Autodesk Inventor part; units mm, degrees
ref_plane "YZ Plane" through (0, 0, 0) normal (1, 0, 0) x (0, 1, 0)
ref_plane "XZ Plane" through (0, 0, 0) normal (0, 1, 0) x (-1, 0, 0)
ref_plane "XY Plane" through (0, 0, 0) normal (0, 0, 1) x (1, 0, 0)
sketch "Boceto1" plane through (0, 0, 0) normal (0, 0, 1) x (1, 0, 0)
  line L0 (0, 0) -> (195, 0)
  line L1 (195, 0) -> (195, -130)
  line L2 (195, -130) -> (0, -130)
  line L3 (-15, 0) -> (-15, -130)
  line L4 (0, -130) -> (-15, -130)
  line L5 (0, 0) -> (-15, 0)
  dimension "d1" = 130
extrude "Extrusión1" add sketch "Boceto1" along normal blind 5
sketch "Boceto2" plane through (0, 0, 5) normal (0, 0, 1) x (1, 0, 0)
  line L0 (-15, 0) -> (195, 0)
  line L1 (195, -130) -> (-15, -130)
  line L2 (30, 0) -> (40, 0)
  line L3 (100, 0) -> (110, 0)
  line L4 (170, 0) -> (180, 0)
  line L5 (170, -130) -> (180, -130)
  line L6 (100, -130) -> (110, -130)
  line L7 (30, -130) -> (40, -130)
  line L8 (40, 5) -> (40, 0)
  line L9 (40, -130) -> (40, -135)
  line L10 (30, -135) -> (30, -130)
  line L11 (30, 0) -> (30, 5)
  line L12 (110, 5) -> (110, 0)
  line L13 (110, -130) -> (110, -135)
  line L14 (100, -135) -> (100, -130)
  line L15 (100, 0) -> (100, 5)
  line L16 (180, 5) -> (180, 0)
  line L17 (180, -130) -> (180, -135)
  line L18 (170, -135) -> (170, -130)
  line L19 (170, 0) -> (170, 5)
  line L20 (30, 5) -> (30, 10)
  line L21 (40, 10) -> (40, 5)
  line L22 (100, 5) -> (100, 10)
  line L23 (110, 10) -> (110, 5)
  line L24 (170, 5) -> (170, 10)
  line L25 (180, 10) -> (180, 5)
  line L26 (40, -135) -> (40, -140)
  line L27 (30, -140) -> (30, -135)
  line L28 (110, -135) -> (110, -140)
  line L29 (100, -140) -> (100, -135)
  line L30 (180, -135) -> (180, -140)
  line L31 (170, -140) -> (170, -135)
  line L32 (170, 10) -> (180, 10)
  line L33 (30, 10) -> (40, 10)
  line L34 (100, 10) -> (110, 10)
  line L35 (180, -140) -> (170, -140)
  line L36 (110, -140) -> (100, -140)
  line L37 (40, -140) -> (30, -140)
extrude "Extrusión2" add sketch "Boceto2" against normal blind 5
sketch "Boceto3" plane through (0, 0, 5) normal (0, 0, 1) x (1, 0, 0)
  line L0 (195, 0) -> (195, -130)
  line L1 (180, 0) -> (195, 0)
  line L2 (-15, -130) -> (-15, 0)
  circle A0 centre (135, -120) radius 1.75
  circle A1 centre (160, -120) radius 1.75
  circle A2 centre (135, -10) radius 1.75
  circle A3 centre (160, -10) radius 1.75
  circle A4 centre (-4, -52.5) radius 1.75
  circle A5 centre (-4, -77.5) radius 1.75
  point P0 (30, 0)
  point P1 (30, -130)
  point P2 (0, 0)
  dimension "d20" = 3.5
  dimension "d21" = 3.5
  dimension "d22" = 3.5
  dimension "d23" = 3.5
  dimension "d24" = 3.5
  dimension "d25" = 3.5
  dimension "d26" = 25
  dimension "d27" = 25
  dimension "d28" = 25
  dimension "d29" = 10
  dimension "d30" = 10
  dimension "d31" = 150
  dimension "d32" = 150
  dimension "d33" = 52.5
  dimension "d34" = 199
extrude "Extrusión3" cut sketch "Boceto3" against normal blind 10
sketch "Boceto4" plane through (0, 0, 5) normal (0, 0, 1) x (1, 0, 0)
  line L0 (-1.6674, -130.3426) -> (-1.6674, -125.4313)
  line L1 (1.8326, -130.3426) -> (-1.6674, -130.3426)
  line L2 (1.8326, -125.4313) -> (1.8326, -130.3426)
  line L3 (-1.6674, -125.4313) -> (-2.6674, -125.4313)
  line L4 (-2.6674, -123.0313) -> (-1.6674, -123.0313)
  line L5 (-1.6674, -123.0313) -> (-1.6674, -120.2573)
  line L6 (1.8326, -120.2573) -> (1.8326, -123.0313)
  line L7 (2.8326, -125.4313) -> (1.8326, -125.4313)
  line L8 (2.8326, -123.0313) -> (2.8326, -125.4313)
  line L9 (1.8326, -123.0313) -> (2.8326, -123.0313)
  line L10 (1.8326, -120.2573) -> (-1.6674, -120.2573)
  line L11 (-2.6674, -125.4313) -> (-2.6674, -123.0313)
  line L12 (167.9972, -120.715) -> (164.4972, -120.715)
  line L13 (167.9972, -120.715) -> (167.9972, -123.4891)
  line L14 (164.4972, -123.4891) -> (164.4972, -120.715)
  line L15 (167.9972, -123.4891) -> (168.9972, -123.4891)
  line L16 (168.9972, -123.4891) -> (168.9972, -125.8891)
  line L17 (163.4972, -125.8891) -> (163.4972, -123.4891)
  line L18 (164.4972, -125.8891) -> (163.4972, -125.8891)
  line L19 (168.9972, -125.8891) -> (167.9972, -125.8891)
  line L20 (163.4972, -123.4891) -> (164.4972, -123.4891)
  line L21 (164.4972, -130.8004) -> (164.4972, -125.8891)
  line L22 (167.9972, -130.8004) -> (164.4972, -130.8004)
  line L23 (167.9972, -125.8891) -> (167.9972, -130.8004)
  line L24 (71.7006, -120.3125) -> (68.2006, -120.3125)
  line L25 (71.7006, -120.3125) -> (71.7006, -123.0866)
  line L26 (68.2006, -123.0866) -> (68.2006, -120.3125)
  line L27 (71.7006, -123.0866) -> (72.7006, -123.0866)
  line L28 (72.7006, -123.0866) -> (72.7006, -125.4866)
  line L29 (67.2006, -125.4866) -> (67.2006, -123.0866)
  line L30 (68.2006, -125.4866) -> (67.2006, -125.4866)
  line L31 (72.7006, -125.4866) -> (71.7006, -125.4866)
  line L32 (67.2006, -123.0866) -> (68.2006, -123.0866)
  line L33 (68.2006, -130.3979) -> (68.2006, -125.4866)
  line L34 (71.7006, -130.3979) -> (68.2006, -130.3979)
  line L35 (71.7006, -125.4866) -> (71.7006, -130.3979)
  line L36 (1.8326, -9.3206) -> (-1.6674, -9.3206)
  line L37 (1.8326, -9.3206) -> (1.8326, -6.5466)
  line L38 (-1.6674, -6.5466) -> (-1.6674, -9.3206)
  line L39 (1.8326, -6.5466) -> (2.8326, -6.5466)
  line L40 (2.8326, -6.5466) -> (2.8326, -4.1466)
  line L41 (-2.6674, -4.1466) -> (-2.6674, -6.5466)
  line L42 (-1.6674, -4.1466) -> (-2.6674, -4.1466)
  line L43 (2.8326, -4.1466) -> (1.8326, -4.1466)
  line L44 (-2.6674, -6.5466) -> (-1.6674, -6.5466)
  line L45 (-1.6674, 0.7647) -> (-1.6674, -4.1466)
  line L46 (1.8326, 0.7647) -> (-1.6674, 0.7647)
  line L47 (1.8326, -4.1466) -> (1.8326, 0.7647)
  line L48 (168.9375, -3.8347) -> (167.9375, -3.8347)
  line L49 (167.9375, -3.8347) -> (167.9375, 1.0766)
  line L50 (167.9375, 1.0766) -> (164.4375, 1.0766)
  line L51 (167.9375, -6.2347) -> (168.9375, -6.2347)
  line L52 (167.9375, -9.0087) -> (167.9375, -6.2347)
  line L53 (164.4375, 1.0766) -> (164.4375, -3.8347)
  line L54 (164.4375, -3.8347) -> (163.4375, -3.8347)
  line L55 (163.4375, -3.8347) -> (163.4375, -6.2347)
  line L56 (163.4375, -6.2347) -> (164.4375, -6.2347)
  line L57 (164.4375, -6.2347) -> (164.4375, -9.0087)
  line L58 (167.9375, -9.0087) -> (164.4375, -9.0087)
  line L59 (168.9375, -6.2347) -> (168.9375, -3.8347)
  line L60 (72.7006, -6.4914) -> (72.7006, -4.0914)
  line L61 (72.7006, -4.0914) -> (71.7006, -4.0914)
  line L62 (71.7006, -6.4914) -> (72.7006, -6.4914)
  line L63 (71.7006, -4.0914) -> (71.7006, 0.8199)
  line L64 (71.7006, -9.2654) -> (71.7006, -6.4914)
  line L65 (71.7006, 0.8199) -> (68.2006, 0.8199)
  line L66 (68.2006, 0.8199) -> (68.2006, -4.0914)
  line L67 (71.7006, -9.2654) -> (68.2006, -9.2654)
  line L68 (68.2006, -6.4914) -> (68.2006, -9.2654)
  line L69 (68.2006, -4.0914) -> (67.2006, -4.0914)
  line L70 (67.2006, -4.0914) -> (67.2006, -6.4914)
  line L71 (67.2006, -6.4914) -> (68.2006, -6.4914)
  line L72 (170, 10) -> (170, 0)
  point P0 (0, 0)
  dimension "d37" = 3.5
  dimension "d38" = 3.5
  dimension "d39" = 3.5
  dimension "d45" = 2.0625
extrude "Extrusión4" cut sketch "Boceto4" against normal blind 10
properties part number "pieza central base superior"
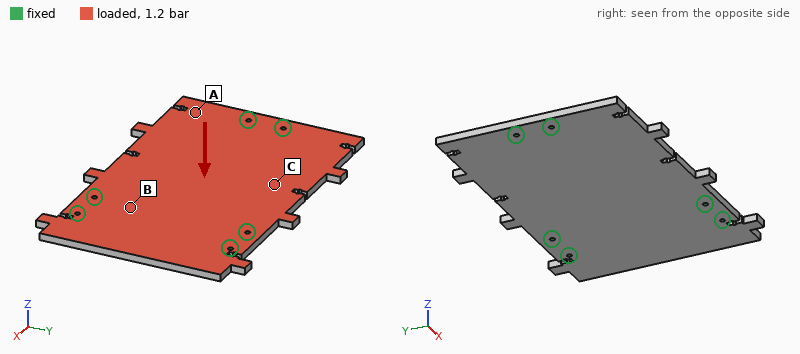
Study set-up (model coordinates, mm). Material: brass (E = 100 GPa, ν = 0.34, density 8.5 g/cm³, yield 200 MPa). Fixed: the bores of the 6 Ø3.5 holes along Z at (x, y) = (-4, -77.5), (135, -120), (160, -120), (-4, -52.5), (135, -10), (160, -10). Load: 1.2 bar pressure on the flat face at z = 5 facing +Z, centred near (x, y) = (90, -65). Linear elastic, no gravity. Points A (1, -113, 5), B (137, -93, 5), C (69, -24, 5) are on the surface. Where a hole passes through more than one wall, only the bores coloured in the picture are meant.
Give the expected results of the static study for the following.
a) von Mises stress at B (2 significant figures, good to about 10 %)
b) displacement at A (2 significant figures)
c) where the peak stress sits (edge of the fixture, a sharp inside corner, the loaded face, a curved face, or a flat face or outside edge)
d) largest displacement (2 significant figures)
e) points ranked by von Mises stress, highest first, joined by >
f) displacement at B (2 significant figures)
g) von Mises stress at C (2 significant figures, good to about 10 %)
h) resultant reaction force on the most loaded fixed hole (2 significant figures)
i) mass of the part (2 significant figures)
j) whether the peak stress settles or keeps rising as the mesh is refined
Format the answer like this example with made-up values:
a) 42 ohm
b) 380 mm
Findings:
a) 23 MPa
b) 0.10 mm
c) edge of the fixture
d) 0.28 mm
e) C > B > A
f) 0.048 mm
g) 34 MPa
h) 780 N
i) 1.2 kg
j) keeps rising
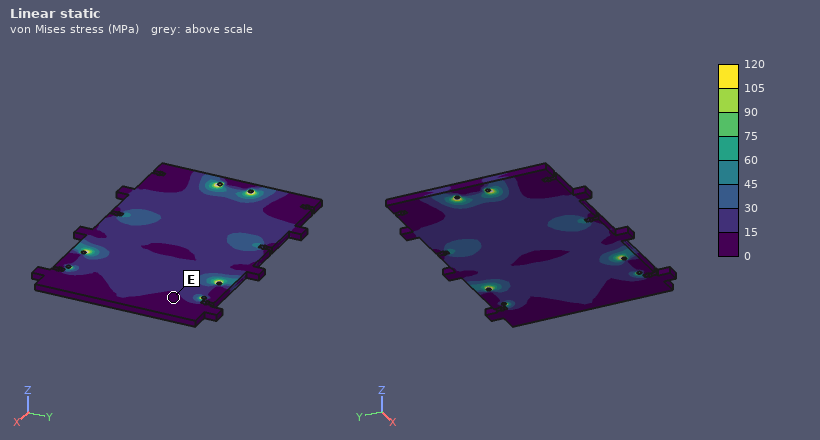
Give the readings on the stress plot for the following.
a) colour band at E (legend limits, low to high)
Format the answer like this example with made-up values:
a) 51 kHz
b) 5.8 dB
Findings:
a) 0 to 15 MPa
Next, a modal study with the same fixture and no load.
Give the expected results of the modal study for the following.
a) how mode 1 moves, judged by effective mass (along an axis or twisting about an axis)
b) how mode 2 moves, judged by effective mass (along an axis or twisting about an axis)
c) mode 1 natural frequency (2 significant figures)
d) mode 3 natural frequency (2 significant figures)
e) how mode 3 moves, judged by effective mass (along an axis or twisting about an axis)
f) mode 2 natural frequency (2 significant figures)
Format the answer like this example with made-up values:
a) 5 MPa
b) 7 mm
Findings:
a) along Z
b) twisting about X
c) 650 Hz
d) 1000 Hz
e) along Z
f) 690 Hz
